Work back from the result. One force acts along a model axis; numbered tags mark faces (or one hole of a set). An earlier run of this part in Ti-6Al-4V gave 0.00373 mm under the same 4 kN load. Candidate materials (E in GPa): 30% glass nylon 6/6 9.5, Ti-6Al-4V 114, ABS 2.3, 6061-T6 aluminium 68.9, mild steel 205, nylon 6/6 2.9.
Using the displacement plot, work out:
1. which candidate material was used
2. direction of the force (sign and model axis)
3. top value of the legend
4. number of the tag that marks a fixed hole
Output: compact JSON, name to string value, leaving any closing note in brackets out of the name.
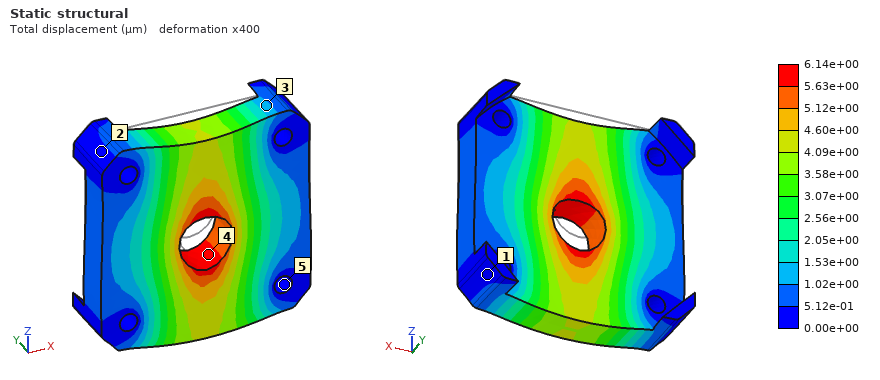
{"which candidate material was used": "6061-T6 aluminium", "direction of the force": "-Z", "top value of the legend": "6.14e+00 µm", "number of the tag that marks a fixed hole": "5"}
